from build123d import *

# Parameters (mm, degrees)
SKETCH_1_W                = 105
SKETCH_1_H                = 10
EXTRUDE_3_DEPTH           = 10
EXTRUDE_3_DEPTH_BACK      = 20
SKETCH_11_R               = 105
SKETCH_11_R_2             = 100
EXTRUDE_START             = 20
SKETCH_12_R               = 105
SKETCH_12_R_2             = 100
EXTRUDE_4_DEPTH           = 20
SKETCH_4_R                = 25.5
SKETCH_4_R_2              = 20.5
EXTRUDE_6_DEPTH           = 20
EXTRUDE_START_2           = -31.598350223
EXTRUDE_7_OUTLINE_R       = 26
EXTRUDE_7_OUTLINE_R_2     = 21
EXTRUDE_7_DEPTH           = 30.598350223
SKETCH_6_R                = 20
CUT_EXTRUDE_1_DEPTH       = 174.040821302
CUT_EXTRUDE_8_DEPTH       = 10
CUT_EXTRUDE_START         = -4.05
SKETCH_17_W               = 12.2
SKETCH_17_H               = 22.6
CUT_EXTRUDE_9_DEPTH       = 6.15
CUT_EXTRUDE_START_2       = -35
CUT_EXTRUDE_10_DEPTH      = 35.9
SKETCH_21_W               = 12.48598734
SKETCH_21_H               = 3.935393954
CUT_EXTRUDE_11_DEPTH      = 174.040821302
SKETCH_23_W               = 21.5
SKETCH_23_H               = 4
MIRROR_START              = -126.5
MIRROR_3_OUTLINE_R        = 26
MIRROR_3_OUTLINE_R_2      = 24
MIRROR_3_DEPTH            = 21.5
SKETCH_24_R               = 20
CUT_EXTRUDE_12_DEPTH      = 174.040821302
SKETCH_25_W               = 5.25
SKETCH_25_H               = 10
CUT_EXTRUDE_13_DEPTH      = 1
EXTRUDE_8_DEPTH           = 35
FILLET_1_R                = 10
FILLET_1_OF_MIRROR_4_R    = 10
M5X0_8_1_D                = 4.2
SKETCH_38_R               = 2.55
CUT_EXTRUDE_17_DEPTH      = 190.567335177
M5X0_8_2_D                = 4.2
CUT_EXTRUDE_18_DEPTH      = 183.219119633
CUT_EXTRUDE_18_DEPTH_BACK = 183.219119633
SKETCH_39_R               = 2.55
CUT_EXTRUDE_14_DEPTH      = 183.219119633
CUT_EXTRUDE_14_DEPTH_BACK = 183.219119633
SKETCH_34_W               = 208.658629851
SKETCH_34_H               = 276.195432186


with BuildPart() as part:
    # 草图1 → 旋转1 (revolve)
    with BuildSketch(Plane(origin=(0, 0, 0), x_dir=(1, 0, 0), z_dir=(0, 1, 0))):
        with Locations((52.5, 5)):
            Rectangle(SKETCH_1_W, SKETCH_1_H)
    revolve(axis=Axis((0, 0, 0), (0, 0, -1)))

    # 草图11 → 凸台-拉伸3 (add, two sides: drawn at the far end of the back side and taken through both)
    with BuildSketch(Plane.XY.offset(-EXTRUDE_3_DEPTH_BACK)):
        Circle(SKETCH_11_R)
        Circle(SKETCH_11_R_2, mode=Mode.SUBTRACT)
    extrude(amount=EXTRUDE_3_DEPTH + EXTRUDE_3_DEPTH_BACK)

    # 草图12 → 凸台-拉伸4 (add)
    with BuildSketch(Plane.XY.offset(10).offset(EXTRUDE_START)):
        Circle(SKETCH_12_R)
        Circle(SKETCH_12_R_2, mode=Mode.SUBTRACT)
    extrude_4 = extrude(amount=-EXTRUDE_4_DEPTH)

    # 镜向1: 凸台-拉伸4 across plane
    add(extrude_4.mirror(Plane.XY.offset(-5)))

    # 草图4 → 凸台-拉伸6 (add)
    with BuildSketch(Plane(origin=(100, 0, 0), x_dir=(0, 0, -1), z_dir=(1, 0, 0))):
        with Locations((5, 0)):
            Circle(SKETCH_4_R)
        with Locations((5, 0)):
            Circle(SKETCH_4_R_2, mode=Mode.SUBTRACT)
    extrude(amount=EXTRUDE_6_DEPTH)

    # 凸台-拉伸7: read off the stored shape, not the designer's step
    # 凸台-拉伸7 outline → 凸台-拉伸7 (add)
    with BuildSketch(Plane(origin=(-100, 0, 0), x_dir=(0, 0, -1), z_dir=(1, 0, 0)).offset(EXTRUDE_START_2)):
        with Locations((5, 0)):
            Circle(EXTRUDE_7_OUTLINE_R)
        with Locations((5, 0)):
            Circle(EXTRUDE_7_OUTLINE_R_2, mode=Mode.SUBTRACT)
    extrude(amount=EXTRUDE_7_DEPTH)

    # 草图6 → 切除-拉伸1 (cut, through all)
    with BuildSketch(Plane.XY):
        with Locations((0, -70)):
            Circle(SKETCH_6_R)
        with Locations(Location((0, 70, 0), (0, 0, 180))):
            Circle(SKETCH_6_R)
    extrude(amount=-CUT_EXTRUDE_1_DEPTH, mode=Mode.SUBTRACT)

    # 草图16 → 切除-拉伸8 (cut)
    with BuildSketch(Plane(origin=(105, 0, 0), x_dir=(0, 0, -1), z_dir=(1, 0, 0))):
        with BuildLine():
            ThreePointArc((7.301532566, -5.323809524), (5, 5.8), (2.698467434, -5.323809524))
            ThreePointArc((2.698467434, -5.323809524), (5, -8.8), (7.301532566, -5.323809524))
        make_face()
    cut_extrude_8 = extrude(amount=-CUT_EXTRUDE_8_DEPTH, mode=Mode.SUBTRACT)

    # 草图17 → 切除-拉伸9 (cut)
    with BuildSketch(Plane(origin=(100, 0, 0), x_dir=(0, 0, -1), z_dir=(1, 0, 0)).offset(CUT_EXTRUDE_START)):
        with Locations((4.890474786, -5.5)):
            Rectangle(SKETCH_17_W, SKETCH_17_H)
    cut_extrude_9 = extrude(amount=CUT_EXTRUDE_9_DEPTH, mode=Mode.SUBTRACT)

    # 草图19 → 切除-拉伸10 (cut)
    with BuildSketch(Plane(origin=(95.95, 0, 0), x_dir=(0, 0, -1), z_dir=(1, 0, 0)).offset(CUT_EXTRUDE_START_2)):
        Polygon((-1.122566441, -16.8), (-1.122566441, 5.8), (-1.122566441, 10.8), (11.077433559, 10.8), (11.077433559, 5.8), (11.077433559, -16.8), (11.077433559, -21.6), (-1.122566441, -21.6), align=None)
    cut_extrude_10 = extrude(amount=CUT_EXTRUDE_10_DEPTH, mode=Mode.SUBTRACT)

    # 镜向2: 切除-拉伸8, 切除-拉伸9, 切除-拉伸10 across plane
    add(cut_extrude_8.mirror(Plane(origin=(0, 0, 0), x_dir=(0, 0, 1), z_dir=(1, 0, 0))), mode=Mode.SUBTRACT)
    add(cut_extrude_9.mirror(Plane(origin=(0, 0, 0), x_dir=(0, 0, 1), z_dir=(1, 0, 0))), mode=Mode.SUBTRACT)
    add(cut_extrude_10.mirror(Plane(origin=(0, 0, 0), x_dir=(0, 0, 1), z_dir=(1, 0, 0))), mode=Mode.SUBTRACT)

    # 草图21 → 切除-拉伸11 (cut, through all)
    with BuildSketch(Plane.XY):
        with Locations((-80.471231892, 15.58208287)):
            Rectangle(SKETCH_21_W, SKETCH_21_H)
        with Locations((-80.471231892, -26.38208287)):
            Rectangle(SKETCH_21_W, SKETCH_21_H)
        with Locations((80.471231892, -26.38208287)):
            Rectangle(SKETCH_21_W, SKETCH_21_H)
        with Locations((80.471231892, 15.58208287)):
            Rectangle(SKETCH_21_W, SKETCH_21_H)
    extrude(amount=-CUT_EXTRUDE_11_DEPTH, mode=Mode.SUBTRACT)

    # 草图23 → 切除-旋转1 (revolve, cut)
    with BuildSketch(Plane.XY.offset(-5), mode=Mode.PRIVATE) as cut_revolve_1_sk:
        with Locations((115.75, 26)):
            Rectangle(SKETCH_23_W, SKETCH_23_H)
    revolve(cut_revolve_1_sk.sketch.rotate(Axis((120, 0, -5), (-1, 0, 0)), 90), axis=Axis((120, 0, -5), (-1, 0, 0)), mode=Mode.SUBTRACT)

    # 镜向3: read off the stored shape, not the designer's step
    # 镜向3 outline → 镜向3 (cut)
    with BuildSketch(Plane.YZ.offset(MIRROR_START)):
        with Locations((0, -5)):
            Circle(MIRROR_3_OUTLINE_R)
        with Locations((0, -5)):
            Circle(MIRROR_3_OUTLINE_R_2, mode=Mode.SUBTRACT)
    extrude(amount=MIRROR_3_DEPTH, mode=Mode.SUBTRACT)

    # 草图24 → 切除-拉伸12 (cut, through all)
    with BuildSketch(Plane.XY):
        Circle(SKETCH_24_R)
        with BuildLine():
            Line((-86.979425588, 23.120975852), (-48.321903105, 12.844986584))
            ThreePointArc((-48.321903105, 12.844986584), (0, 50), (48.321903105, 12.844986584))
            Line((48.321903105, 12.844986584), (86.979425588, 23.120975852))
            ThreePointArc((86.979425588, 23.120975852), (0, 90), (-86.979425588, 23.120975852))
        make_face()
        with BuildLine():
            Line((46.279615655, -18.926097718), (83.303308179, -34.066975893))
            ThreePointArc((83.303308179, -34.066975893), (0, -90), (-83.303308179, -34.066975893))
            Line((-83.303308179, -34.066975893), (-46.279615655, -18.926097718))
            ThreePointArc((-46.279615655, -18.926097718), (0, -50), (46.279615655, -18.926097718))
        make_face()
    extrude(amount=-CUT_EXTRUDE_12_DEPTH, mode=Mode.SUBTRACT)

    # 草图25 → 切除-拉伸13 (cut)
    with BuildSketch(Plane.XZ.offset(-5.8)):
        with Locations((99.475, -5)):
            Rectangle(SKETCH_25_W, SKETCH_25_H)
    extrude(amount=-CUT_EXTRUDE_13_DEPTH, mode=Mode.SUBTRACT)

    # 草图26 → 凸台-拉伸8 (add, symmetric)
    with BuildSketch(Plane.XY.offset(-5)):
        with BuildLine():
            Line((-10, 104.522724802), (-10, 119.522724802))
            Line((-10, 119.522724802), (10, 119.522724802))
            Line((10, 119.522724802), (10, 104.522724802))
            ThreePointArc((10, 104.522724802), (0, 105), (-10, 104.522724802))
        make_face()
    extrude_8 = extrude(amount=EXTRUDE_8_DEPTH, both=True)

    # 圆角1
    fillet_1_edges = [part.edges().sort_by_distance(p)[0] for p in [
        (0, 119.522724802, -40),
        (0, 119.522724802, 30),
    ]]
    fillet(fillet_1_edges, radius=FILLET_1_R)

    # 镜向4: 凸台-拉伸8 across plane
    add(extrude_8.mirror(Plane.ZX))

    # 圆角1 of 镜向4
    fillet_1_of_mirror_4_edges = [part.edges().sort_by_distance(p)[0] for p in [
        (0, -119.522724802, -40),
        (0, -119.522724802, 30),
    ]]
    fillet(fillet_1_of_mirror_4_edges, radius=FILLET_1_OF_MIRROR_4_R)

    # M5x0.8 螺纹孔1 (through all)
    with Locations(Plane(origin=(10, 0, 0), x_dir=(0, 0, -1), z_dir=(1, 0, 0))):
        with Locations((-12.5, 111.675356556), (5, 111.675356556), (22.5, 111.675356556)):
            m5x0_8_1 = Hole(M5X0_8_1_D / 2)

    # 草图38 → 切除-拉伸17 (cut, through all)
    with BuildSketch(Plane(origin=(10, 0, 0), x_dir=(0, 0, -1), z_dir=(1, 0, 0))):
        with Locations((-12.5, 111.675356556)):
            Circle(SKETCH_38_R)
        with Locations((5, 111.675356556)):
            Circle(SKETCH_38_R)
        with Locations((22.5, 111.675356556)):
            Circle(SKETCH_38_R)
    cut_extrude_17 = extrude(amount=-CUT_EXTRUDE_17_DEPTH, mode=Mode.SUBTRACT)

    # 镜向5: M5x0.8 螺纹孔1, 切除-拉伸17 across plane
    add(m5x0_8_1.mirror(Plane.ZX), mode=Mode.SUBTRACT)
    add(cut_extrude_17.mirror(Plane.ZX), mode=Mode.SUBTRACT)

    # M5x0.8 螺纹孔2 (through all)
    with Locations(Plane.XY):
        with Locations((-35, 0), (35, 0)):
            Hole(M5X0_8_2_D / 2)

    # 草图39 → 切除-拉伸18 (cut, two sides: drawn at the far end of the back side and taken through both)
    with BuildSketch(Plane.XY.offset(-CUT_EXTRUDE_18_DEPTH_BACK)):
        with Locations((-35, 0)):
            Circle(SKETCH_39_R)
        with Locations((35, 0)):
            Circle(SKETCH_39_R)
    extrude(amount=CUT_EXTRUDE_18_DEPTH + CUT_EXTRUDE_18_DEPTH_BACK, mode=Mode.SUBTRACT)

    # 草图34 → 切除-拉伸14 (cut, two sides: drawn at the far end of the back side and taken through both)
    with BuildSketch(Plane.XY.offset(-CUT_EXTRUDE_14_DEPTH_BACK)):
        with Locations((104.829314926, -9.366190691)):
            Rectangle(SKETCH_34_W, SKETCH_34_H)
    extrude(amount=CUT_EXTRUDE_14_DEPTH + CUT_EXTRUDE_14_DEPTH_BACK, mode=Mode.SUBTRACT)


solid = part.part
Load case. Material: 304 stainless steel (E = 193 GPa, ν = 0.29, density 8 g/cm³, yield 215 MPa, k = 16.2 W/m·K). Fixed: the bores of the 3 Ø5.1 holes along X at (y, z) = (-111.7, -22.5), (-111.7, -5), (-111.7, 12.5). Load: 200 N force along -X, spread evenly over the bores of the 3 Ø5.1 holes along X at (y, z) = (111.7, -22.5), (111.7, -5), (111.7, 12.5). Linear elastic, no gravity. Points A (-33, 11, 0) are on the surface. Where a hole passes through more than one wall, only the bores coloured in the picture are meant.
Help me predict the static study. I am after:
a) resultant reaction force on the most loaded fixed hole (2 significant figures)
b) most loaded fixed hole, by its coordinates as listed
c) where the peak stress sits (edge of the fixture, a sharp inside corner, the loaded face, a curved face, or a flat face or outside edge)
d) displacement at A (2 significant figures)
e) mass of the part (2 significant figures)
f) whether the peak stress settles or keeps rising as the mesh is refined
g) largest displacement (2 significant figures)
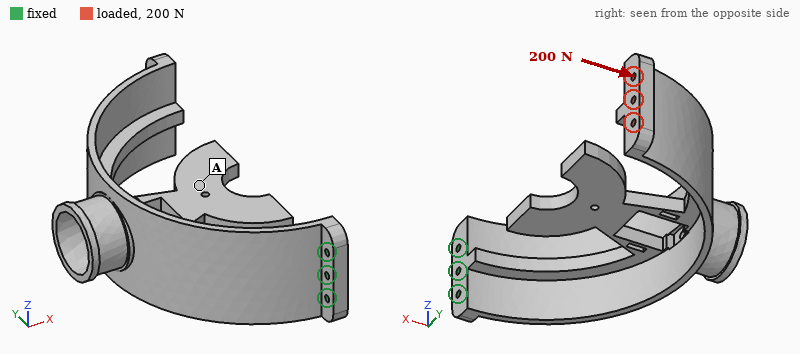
840 N
(-111.7, -5)
edge of the fixture
0.51 mm
1.7 kg
keeps rising
1.3 mm
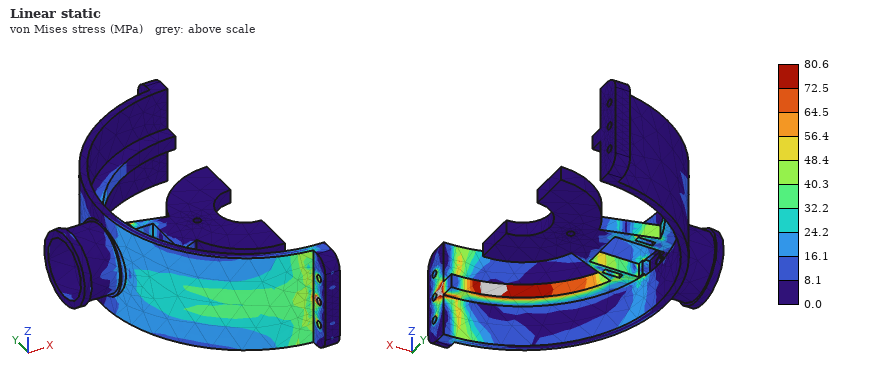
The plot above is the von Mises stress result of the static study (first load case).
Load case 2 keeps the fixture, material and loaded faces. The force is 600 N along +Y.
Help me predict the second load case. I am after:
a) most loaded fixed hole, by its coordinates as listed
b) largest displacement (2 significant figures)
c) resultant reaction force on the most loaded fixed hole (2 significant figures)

(-111.7, -5)
1.5 mm
480 N
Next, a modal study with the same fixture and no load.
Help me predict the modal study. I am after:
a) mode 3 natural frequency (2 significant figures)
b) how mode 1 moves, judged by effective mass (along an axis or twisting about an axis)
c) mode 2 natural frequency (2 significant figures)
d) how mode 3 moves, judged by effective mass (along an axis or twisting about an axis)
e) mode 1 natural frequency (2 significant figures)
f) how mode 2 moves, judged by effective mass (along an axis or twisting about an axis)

270 Hz
along Z
90 Hz
along Y
85 Hz
along X
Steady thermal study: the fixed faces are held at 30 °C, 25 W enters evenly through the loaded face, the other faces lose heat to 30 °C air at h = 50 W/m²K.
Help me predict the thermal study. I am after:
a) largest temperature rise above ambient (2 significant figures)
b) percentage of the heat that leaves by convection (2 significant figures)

80 K
100 %
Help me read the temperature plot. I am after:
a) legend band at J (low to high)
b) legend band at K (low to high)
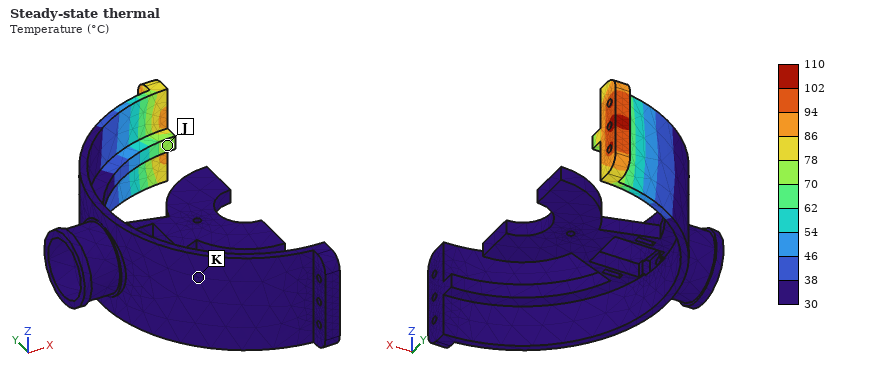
70 to 78 °C
30 to 38 °C
